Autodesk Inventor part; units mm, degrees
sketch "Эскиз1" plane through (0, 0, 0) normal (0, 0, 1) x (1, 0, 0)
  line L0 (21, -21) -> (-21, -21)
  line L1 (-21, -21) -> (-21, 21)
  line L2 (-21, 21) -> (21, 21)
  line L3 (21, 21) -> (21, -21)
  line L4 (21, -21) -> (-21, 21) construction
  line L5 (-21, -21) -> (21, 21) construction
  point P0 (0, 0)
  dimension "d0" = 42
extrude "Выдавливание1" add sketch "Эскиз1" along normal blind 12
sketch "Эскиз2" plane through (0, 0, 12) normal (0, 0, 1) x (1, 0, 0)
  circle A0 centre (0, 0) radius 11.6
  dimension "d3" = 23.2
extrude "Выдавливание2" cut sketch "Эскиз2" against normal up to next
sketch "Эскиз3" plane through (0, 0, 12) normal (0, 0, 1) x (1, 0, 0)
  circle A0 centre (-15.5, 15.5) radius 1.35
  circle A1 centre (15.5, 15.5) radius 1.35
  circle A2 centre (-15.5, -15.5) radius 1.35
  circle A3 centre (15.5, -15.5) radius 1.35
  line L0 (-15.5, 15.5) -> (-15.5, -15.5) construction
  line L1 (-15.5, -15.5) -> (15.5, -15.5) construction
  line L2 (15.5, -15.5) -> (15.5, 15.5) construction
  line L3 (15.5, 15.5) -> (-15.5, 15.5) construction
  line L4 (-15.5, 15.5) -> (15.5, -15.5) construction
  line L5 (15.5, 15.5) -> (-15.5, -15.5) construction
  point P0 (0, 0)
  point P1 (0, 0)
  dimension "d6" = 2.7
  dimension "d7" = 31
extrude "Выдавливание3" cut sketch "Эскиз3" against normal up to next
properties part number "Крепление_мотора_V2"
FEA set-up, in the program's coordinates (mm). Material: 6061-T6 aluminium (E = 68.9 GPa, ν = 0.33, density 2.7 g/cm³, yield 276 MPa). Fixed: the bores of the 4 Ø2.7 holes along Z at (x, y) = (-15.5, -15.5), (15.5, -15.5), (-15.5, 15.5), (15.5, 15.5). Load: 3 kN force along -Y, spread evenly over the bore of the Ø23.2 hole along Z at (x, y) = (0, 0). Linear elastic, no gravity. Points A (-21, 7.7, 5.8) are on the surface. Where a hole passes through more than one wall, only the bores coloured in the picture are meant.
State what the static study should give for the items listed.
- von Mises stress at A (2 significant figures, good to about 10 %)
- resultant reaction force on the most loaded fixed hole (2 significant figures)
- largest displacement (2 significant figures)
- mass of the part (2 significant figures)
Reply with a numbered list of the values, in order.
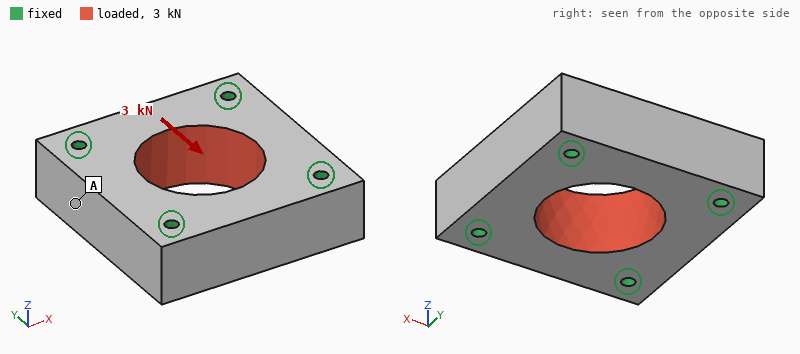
1. 4.1 MPa
2. 770 N
3. 2.6 µm
4. 43 g
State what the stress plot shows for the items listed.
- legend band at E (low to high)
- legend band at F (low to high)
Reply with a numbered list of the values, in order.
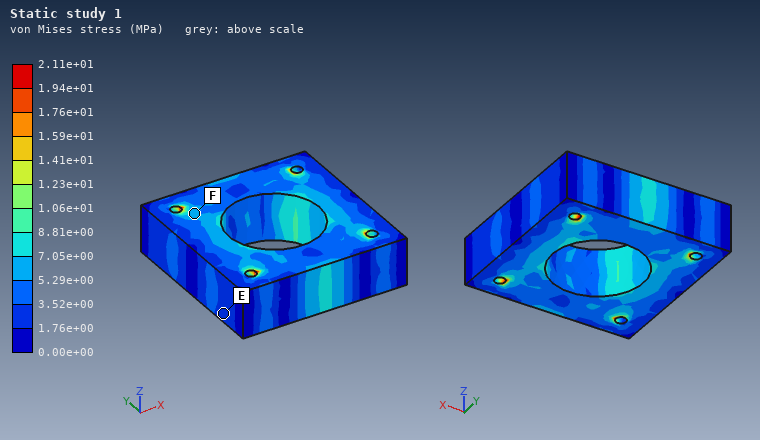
1. 1.76e+00 to 3.52e+00 MPa
2. 5.29e+00 to 7.05e+00 MPa
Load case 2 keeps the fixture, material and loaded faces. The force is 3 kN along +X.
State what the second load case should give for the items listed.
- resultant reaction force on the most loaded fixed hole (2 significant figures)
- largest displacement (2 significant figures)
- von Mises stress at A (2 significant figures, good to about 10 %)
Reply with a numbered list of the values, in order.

1. 770 N
2. 2.6 µm
3. 2.9 MPa
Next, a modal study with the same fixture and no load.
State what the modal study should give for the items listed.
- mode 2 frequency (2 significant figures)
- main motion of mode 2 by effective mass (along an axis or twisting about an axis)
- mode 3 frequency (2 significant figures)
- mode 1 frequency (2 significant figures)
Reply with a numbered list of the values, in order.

1. 34 kHz
2. along Z
3. 37 kHz
4. 26 kHz
